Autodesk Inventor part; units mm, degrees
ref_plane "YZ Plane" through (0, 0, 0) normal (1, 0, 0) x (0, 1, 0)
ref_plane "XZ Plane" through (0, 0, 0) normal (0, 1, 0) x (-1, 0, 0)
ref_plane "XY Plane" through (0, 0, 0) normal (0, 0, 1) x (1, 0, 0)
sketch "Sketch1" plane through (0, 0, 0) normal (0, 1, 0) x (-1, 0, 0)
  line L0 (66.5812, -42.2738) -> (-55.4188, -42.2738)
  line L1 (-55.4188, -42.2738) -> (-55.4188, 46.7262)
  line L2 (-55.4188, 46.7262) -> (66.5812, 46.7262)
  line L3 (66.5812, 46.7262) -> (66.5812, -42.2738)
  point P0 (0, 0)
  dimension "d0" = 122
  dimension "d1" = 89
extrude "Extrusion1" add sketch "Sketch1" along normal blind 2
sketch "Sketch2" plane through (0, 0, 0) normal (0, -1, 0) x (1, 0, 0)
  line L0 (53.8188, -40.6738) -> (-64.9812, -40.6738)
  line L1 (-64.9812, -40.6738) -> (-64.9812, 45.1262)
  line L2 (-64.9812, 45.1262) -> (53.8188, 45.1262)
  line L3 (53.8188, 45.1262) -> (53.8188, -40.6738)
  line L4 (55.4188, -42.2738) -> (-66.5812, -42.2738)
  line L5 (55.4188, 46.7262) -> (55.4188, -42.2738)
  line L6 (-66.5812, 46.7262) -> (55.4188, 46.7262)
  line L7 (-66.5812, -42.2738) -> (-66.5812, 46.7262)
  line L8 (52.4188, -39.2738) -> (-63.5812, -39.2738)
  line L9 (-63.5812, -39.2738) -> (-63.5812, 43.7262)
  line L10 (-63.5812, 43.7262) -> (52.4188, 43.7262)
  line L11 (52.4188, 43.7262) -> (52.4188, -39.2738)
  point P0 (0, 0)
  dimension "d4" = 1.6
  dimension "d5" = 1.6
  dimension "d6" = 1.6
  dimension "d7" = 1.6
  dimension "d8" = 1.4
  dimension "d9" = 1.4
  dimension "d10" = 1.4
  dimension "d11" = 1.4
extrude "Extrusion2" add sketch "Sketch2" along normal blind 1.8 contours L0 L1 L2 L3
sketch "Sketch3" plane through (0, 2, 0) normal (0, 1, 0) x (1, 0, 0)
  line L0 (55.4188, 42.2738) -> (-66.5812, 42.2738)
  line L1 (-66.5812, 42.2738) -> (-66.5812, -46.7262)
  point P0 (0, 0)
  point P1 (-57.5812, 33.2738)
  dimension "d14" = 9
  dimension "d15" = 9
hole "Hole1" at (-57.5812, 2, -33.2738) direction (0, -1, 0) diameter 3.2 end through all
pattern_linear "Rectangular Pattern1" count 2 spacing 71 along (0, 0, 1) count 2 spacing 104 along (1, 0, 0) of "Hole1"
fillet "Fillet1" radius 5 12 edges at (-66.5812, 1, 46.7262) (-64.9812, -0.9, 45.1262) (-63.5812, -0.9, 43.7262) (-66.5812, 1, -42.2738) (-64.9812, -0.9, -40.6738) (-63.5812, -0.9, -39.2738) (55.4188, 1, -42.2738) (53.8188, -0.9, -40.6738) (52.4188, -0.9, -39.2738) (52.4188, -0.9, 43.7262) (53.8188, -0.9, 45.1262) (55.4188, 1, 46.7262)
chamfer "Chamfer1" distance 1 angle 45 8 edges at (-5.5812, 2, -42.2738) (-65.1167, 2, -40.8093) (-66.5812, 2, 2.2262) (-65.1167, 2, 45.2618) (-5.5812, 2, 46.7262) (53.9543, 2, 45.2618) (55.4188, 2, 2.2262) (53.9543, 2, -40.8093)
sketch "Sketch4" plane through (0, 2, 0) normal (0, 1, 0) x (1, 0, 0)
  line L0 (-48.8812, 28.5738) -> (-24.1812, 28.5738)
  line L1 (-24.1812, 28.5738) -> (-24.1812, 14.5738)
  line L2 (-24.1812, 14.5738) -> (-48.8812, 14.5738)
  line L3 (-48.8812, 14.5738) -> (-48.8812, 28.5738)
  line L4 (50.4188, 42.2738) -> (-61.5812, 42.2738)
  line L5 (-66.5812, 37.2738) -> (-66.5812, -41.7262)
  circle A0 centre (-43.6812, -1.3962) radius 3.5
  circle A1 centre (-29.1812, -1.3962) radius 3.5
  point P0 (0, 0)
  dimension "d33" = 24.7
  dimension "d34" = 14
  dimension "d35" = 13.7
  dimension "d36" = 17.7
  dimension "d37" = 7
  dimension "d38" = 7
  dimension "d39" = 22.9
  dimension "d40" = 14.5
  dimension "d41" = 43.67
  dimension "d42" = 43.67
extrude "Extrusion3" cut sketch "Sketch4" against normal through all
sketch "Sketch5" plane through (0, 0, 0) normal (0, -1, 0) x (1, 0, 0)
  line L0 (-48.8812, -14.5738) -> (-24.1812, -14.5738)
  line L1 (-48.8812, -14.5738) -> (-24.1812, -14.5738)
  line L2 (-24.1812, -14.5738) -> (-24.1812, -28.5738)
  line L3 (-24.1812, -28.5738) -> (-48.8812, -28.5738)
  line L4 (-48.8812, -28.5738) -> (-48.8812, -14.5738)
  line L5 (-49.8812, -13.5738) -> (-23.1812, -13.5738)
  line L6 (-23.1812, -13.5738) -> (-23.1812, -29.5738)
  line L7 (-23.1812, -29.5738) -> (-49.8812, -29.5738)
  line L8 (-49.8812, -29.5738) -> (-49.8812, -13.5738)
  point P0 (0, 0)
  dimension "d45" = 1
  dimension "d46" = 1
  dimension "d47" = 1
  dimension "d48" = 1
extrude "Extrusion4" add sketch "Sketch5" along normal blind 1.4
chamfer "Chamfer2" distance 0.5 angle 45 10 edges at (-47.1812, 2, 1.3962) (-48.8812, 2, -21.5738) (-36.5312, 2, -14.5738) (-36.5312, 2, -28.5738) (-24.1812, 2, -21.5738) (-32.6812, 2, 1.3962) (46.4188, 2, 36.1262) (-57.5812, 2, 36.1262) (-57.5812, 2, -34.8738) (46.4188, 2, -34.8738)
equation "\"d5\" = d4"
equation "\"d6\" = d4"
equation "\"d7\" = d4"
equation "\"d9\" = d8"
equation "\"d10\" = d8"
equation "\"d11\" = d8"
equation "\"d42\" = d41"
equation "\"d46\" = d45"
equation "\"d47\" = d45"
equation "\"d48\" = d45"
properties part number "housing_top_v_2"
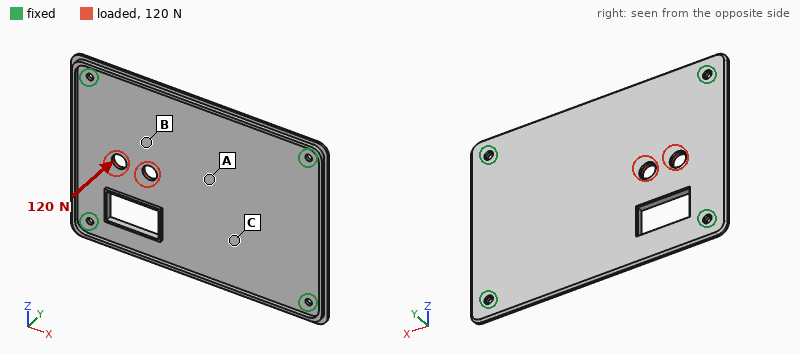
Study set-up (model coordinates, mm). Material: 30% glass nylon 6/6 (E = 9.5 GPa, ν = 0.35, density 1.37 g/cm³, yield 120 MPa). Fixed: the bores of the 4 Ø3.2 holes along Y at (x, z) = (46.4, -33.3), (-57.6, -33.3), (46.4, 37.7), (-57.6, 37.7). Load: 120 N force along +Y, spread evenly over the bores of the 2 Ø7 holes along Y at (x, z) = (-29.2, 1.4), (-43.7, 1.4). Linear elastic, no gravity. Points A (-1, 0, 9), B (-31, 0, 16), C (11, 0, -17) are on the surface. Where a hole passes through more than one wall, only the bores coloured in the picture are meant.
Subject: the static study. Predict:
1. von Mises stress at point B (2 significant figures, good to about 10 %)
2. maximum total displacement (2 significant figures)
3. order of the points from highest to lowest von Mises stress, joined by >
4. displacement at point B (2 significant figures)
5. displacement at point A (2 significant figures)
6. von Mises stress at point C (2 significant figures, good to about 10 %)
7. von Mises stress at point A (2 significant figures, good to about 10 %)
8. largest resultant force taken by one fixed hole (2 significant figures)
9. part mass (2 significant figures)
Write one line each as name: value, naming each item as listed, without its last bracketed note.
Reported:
von Mises stress at point B: 17 MPa
maximum total displacement: 1.5 mm
order of the points from highest to lowest von Mises stress, joined by >: B > A > C
displacement at point B: 1.1 mm
displacement at point A: 0.97 mm
von Mises stress at point C: 5.4 MPa
von Mises stress at point A: 9.7 MPa
largest resultant force taken by one fixed hole: 52 N
part mass: 30 g
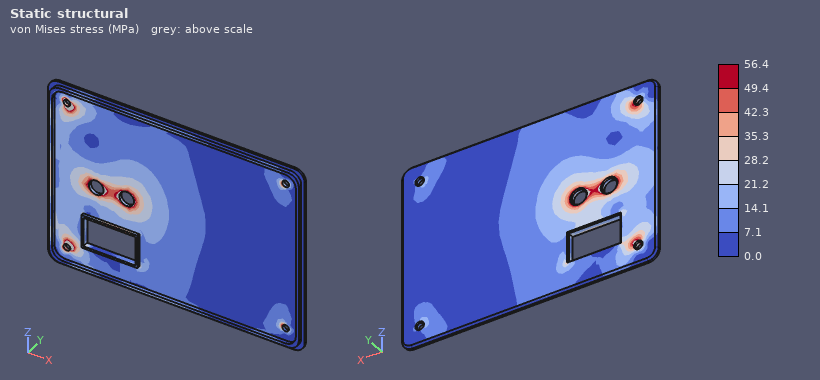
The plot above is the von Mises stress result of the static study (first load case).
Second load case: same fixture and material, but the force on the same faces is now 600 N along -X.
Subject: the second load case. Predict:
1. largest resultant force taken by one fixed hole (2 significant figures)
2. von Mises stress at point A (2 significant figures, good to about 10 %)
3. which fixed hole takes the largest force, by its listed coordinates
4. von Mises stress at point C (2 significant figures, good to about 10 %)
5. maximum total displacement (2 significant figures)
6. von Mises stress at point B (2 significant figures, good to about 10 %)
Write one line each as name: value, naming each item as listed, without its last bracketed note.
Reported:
largest resultant force taken by one fixed hole: 200 N
von Mises stress at point A: 3.8 MPa
which fixed hole takes the largest force, by its listed coordinates: (-57.6, 37.7)
von Mises stress at point C: 2.4 MPa
maximum total displacement: 68 µm
von Mises stress at point B: 4.5 MPa
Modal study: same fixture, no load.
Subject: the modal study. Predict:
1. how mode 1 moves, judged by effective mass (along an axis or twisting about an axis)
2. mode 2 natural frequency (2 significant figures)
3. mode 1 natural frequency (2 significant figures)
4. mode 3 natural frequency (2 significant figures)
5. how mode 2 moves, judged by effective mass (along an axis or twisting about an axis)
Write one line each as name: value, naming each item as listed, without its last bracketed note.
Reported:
how mode 1 moves, judged by effective mass: along Y
mode 2 natural frequency: 680 Hz
mode 1 natural frequency: 440 Hz
mode 3 natural frequency: 990 Hz
how mode 2 moves, judged by effective mass: twisting about X
